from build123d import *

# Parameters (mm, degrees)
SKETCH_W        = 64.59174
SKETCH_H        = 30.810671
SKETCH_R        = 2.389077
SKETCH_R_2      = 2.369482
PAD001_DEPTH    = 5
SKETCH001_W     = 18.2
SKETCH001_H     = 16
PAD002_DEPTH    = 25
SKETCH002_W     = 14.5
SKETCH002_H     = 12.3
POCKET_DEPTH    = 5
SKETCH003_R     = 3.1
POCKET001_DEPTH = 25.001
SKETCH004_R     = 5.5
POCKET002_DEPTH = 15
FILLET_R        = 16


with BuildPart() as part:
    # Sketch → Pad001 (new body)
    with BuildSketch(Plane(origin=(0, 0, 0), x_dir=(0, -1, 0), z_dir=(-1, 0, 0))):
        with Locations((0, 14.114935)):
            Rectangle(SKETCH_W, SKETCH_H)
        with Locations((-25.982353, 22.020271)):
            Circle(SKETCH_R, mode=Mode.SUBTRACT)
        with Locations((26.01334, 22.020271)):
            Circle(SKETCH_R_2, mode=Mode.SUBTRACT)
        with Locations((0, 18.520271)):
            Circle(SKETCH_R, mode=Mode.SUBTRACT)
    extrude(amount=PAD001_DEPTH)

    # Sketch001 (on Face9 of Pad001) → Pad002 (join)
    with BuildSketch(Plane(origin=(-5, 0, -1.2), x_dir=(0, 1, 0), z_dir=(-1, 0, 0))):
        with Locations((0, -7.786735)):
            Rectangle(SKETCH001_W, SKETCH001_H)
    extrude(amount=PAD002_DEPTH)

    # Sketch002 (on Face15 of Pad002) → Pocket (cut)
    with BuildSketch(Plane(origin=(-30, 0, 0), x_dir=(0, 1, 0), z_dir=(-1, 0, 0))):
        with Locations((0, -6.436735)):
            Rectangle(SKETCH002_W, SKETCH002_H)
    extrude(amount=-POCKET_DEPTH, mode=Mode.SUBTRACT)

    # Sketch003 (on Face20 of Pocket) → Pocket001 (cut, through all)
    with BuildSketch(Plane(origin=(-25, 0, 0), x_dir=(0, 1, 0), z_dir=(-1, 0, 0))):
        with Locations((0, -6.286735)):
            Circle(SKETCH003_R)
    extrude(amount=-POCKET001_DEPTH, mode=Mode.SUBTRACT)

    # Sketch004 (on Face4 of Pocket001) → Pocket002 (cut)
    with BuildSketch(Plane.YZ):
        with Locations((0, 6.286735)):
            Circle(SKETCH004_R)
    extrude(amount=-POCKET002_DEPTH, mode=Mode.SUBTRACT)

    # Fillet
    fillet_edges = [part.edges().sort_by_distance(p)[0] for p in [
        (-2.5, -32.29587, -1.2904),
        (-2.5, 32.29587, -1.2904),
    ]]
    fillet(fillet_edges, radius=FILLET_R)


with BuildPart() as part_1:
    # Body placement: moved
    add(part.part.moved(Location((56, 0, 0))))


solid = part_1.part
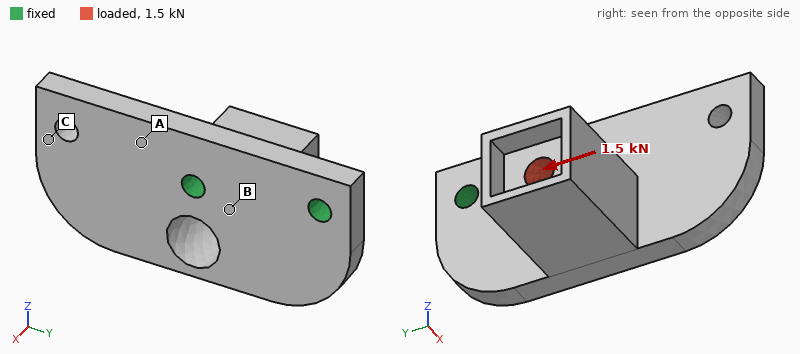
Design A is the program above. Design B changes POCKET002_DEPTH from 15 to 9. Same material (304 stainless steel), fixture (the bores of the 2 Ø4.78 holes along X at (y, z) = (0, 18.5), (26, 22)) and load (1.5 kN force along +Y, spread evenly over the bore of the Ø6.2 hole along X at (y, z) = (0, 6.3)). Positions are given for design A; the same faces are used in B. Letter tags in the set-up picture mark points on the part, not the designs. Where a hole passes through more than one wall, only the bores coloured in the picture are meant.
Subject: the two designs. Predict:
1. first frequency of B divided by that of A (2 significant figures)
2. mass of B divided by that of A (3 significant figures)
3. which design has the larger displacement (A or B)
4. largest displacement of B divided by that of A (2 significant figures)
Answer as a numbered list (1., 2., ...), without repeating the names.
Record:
1. 0.99
2. 1.03
3. A
4. 0.80
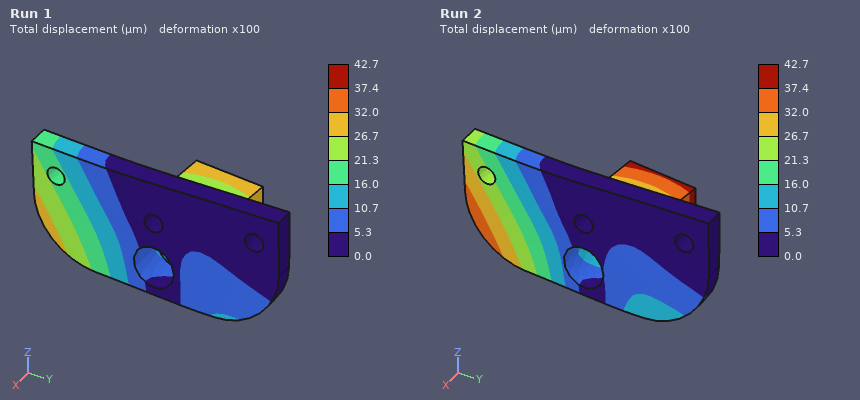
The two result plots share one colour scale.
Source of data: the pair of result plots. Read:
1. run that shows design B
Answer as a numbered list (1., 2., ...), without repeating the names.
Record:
1. Run 1
